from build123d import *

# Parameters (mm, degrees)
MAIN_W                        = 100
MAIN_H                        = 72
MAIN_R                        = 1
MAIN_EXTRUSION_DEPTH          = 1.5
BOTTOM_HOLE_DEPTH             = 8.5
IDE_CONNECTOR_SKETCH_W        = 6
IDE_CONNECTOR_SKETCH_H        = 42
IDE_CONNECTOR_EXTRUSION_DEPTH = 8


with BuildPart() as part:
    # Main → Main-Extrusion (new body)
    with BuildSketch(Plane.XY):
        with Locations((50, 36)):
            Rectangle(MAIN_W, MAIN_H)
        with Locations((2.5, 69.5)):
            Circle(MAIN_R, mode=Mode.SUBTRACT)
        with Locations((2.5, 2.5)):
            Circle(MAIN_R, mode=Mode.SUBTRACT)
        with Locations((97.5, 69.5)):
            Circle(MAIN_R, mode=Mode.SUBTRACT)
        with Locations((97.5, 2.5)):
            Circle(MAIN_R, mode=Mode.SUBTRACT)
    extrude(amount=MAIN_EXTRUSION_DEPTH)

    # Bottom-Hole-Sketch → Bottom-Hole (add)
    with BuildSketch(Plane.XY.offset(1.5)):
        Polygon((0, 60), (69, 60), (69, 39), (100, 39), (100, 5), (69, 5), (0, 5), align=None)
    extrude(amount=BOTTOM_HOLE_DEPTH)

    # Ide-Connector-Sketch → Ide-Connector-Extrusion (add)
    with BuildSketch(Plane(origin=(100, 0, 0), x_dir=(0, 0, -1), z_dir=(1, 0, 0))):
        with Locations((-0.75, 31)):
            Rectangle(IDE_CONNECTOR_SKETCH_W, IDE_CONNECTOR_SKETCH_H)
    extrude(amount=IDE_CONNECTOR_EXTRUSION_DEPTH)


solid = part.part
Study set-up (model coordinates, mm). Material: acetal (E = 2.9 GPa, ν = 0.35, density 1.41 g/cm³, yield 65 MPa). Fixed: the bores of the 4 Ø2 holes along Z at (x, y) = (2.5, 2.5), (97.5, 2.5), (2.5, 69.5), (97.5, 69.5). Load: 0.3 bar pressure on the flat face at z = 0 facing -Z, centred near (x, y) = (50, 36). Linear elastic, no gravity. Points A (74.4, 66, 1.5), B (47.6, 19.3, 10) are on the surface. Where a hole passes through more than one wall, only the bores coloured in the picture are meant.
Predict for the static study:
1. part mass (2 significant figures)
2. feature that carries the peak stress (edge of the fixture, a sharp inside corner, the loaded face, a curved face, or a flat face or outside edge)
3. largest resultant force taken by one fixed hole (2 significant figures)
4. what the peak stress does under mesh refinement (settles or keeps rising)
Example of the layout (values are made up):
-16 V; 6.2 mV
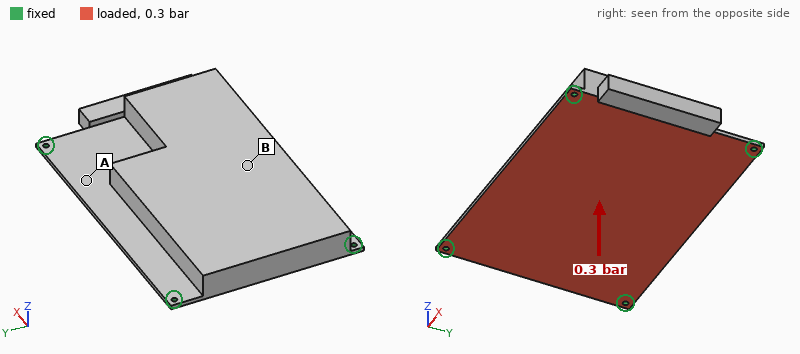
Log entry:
76 g; edge of the fixture; 130 N; keeps rising
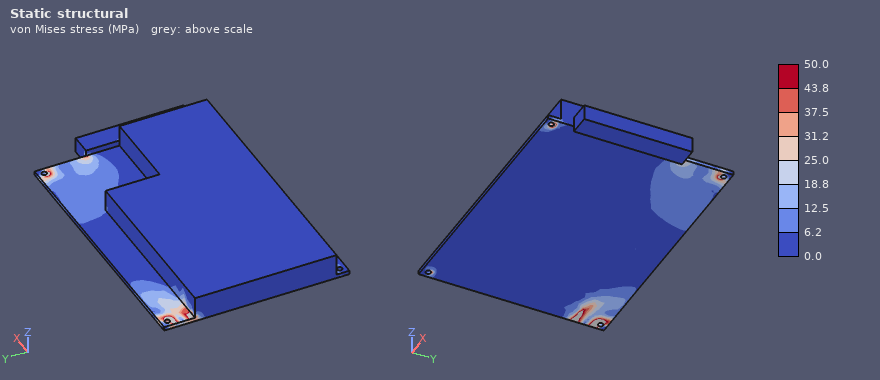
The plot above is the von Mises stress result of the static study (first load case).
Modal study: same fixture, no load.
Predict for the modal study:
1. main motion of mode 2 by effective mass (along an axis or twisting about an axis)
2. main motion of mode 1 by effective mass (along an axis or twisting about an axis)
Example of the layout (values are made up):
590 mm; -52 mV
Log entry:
twisting about Y; along Z
